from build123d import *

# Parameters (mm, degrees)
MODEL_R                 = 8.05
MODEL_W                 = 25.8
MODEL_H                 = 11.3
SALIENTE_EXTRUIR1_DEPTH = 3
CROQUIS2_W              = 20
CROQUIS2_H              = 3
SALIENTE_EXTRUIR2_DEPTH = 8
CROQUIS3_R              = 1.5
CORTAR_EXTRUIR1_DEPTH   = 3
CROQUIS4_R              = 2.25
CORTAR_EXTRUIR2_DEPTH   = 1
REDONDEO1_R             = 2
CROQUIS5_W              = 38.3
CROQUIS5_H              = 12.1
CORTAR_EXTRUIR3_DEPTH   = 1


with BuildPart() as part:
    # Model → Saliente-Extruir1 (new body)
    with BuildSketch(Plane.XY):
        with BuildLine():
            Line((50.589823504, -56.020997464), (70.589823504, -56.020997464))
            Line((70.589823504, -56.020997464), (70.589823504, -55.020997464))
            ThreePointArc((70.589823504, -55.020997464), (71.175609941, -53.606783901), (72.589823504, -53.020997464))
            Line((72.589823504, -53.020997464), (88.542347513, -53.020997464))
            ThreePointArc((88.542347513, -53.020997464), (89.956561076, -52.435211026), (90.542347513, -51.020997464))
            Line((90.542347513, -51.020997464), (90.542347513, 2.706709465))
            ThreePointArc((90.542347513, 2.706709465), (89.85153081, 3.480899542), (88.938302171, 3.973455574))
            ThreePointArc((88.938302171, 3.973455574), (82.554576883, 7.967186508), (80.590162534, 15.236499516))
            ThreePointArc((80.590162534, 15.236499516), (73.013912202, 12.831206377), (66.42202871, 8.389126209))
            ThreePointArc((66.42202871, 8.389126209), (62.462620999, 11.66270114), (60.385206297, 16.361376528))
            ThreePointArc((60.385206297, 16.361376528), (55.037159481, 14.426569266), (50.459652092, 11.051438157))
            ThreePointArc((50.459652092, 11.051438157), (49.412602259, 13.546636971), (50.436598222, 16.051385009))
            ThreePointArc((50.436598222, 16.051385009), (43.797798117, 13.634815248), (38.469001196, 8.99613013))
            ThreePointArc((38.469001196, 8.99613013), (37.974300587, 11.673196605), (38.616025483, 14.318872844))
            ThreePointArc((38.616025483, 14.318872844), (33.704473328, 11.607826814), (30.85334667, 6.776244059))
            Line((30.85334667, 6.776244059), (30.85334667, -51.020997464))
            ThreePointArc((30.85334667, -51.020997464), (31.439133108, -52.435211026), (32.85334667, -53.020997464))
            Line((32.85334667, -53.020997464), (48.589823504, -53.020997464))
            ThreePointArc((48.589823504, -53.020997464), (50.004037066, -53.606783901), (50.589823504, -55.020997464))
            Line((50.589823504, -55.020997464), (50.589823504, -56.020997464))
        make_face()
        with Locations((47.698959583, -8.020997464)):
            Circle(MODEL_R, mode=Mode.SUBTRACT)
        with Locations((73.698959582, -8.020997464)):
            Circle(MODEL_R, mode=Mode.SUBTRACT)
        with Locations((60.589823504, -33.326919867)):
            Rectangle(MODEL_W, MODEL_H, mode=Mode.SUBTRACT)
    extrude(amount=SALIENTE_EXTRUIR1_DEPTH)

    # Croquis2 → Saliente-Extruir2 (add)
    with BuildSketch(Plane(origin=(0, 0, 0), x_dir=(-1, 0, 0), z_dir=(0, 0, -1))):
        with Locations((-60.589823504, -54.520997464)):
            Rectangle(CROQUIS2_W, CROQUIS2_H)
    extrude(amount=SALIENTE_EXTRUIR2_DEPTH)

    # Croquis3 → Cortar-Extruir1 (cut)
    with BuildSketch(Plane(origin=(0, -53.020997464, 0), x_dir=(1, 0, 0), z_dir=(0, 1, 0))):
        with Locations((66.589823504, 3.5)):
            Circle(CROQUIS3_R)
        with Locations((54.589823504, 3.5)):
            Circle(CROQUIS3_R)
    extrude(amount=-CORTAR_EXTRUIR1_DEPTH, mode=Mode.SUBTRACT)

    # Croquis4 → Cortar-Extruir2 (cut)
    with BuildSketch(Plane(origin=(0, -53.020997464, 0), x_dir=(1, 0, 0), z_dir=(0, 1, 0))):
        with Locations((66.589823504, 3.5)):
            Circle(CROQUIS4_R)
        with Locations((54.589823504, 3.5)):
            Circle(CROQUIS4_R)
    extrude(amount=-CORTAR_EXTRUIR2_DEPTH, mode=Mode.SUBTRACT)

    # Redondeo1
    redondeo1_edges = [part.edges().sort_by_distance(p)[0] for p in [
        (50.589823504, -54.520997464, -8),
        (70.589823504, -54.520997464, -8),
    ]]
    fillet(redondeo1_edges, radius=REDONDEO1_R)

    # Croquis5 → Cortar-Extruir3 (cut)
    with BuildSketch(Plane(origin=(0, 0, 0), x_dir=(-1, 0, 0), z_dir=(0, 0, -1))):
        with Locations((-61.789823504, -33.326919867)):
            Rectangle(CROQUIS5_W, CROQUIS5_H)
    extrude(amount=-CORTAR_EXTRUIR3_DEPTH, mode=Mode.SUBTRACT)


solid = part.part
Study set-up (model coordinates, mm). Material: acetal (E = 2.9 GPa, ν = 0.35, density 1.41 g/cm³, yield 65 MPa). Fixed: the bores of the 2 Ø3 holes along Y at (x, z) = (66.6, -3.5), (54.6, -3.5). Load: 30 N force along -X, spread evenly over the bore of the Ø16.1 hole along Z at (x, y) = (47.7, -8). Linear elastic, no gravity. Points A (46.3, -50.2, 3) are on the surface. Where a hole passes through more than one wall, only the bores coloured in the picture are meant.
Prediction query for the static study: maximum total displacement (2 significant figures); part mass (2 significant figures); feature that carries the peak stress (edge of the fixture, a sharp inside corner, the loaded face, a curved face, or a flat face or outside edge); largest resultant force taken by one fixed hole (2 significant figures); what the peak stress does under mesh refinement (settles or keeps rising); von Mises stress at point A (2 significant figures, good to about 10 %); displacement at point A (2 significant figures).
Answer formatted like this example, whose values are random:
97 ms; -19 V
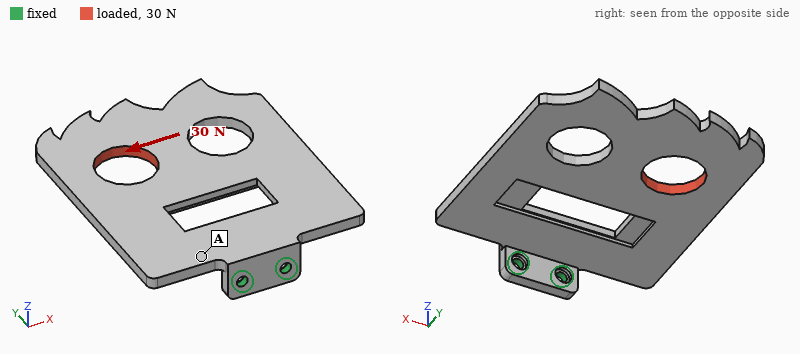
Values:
0.92 mm; 14 g; edge of the fixture; 110 N; keeps rising; 2.3 MPa; 0.18 mm
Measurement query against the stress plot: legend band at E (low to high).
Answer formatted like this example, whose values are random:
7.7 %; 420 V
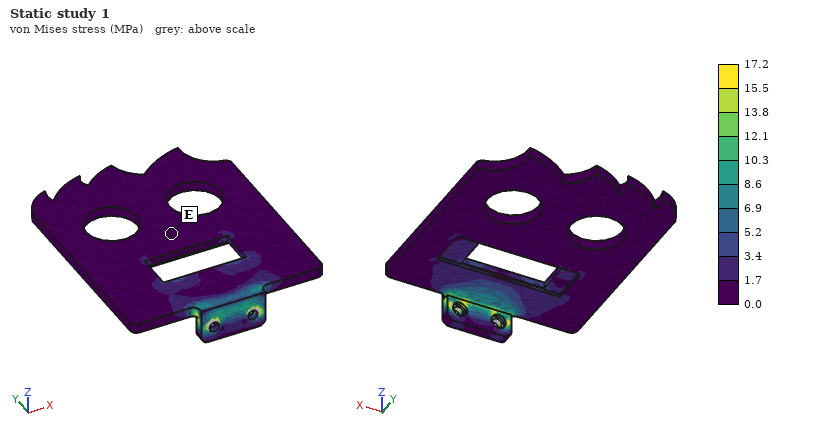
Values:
0.0 to 1.7 MPa
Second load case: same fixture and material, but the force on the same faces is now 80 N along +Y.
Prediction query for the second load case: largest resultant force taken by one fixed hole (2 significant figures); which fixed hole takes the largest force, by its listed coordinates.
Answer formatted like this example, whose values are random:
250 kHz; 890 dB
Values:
120 N; (54.6, -3.5)
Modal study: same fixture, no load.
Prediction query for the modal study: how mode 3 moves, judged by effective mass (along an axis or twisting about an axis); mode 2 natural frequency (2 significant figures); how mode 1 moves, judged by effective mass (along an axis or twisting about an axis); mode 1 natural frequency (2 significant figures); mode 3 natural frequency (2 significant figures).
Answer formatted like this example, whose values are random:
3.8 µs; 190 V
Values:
along X; 260 Hz; along Z; 93 Hz; 370 Hz
